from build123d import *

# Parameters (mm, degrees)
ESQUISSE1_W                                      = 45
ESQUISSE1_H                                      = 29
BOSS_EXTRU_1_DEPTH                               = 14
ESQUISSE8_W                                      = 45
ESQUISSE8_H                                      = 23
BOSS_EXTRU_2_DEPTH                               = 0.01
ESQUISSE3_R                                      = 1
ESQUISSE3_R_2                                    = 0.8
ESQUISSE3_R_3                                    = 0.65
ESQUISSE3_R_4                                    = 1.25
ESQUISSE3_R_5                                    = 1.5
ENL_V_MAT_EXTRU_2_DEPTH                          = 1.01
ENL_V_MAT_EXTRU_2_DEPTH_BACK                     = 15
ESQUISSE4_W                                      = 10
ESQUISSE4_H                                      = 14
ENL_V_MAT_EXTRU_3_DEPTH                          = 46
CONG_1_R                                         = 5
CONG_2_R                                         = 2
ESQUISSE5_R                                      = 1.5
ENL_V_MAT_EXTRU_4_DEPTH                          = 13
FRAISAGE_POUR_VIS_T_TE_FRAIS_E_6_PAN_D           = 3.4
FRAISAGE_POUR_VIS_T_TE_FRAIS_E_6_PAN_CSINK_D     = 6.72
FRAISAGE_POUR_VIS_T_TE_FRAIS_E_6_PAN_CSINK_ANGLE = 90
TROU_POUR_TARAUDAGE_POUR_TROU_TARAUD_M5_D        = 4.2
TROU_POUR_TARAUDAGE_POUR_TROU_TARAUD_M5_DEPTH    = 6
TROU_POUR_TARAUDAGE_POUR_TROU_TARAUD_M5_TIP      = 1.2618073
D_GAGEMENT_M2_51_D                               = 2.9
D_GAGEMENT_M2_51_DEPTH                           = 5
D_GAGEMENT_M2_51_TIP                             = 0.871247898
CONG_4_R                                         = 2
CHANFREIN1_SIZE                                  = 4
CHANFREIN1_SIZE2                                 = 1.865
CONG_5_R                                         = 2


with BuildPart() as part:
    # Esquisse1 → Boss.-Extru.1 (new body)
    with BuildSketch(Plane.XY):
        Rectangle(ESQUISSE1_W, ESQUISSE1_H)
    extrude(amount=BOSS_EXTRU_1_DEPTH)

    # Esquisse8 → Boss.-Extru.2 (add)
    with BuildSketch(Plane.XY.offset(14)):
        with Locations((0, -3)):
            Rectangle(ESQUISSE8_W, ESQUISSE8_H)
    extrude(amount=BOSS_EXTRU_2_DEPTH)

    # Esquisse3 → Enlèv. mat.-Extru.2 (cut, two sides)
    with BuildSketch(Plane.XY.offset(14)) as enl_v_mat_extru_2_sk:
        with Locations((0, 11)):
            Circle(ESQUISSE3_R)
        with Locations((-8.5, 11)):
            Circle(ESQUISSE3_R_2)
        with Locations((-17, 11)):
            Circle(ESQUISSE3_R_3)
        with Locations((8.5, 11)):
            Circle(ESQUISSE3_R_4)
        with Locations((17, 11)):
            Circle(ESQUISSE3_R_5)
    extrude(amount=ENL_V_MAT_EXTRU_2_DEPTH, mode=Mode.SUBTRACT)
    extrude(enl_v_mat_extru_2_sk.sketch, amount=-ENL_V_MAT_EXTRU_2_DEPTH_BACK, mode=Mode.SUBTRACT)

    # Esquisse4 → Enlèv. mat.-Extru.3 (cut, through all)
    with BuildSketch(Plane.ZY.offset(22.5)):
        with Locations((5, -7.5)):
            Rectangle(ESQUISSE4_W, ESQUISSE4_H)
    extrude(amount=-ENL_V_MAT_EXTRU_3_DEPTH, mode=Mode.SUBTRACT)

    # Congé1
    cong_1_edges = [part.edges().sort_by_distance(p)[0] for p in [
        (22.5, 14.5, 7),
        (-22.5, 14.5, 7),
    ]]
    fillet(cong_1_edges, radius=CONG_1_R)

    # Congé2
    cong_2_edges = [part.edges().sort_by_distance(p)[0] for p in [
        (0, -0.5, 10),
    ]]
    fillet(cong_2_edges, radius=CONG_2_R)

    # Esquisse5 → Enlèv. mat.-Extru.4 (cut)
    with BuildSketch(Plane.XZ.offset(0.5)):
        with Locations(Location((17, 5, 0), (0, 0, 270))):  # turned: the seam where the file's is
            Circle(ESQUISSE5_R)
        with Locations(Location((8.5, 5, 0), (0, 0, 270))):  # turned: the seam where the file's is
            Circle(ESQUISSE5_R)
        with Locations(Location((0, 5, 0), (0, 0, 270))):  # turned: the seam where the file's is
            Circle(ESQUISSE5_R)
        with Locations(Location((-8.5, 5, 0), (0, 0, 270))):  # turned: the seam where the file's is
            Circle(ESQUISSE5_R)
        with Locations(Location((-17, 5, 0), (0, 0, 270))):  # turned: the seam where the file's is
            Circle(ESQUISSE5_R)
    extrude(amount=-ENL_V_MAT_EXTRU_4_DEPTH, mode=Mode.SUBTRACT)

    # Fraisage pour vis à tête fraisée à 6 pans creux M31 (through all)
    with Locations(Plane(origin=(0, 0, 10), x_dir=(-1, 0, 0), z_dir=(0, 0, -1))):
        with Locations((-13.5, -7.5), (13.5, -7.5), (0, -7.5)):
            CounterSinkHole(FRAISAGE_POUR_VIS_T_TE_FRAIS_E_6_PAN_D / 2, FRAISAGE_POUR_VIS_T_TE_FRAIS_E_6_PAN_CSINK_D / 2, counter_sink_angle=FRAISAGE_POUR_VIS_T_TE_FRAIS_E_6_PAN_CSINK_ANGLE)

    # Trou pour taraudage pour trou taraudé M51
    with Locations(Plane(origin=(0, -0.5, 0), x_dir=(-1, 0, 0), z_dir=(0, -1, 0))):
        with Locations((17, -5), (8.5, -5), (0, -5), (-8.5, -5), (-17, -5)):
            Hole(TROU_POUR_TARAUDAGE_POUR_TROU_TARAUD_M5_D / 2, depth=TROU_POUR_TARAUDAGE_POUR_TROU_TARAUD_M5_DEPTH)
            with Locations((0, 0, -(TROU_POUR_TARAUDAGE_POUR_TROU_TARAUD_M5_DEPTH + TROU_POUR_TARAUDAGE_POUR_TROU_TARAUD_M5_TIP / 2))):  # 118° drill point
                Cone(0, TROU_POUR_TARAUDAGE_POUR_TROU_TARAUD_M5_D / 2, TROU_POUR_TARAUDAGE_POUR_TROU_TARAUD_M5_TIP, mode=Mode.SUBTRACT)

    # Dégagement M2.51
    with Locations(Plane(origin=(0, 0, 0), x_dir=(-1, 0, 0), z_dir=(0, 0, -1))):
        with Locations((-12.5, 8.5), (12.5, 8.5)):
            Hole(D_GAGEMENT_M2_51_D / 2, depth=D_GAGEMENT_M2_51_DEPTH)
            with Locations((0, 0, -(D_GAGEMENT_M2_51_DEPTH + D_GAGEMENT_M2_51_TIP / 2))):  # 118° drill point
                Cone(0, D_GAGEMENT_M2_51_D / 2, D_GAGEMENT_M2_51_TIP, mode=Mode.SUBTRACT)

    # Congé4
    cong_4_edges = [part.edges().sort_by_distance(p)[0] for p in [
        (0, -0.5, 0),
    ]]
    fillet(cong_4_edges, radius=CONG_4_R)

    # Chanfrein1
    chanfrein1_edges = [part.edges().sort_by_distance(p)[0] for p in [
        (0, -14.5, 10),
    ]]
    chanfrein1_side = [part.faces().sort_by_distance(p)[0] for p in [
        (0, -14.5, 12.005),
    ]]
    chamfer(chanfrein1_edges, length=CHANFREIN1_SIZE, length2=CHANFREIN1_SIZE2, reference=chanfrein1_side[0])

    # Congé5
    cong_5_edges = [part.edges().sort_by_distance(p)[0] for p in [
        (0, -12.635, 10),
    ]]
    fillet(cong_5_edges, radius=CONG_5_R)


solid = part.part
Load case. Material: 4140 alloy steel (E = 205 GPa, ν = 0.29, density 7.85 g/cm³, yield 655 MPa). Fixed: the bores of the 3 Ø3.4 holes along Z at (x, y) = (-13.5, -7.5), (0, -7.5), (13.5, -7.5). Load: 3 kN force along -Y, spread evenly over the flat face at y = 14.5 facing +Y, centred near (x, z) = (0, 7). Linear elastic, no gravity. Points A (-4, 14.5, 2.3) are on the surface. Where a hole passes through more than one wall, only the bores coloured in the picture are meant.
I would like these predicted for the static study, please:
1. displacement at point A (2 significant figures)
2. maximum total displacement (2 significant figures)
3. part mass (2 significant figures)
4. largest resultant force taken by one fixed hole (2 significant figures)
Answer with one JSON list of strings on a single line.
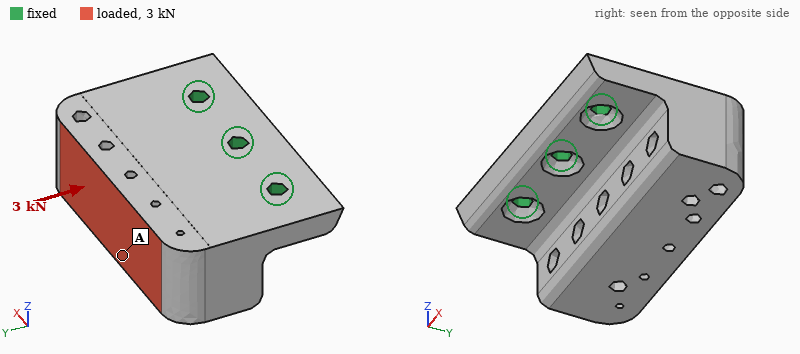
["72 µm", "76 µm", "83 g", "1.1 kN"]
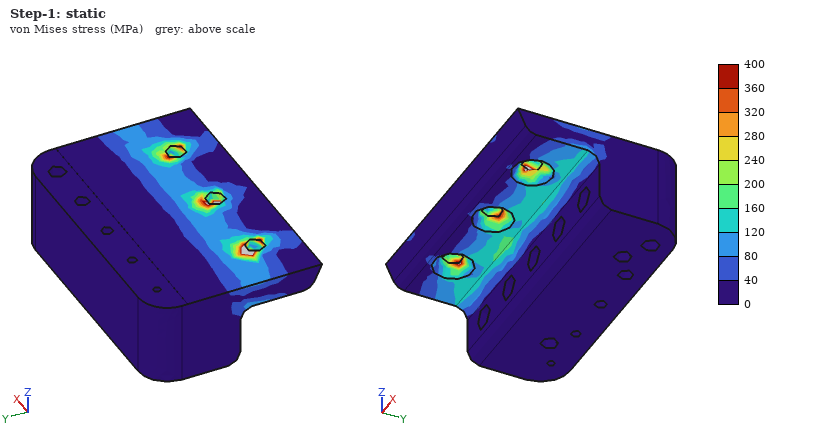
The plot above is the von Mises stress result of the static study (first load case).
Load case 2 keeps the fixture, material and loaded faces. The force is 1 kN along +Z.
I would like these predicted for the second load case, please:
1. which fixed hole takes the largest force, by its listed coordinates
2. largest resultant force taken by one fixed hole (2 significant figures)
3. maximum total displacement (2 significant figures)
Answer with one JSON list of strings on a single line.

["(0, -7.5)", "390 N", "92 µm"]
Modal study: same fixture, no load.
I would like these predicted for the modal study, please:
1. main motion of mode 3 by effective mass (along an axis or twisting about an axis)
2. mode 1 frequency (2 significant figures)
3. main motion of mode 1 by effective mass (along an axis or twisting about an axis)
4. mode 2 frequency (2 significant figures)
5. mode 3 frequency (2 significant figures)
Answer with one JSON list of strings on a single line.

["along X", "3000 Hz", "along Z", "8700 Hz", "15 kHz"]
